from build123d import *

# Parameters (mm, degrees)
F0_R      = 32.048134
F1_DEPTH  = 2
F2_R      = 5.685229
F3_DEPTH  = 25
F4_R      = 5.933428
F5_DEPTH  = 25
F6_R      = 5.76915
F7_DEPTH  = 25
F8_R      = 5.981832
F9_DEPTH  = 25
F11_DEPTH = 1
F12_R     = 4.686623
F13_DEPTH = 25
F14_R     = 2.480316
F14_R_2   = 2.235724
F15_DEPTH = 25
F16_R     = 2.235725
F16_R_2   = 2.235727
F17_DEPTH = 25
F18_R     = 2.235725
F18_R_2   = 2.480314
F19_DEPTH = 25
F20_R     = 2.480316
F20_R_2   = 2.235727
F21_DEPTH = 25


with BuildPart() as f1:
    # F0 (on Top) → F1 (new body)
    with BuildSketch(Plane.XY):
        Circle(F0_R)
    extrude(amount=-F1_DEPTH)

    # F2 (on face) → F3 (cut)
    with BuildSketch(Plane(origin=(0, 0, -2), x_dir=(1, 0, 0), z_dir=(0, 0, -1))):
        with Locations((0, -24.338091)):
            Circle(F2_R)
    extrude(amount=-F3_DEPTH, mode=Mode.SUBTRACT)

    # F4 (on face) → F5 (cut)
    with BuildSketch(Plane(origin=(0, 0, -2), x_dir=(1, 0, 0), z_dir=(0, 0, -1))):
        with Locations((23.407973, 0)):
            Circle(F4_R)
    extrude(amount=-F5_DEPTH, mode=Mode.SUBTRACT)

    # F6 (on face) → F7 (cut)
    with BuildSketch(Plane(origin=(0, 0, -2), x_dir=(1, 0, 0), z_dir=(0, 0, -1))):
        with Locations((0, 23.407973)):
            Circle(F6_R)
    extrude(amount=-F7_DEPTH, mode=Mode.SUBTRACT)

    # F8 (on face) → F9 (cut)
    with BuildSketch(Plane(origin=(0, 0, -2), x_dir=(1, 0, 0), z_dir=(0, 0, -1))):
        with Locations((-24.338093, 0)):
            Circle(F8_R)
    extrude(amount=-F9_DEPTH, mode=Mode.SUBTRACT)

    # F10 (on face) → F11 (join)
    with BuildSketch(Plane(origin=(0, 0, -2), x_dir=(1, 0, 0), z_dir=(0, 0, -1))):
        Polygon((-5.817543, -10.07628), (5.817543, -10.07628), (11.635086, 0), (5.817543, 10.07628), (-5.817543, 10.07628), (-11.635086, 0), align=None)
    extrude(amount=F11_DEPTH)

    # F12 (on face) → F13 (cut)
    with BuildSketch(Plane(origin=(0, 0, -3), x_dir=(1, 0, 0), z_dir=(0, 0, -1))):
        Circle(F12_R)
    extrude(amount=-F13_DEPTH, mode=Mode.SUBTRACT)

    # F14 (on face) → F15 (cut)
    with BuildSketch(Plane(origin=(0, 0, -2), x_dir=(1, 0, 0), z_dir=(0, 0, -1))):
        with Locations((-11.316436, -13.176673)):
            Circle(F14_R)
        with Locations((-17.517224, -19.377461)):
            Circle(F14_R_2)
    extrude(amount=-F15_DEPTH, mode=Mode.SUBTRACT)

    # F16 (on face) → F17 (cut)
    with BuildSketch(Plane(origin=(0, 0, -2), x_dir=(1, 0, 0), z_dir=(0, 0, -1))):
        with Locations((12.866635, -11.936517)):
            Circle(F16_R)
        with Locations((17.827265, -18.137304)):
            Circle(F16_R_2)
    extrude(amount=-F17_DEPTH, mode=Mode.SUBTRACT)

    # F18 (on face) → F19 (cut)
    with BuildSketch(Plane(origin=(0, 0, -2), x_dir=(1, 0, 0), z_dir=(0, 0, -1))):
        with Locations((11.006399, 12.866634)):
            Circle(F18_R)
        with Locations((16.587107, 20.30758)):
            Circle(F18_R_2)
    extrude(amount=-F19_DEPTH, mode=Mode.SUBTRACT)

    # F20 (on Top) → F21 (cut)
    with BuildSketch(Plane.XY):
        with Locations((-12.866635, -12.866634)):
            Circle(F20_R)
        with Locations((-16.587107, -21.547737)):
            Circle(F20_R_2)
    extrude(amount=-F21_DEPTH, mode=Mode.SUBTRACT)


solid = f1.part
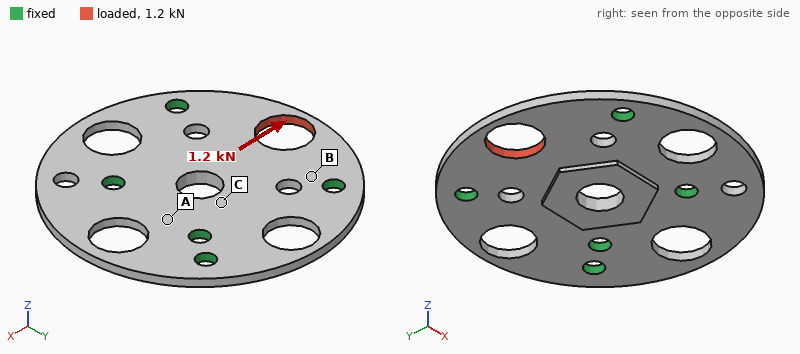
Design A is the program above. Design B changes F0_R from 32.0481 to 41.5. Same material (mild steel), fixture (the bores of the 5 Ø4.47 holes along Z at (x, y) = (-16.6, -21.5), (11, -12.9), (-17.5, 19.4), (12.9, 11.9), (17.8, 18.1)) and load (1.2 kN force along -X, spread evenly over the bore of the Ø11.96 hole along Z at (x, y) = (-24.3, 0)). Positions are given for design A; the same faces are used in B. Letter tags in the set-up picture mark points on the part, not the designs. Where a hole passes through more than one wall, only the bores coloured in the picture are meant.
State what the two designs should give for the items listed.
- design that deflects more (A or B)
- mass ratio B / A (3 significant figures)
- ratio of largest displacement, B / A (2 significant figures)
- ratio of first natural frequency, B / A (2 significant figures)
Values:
A
1.80
0.41
0.41
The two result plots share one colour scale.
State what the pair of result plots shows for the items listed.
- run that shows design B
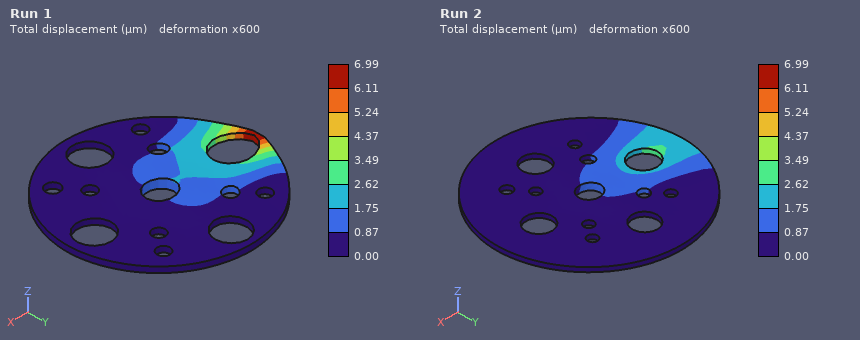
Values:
Run 2
